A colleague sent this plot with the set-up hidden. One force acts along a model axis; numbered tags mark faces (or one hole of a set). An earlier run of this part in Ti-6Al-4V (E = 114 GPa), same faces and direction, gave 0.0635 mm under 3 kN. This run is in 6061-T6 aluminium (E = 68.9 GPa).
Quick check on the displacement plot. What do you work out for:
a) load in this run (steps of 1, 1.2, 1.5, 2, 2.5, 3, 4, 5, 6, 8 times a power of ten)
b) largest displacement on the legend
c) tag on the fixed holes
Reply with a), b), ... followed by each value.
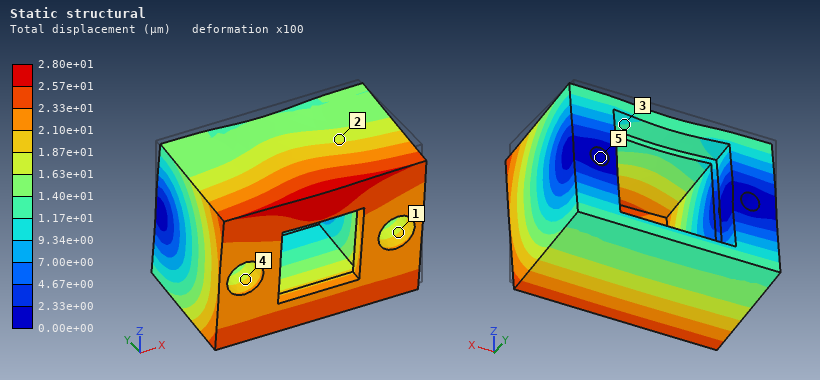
a) 800 N
b) 2.80e+01 µm
c) 5
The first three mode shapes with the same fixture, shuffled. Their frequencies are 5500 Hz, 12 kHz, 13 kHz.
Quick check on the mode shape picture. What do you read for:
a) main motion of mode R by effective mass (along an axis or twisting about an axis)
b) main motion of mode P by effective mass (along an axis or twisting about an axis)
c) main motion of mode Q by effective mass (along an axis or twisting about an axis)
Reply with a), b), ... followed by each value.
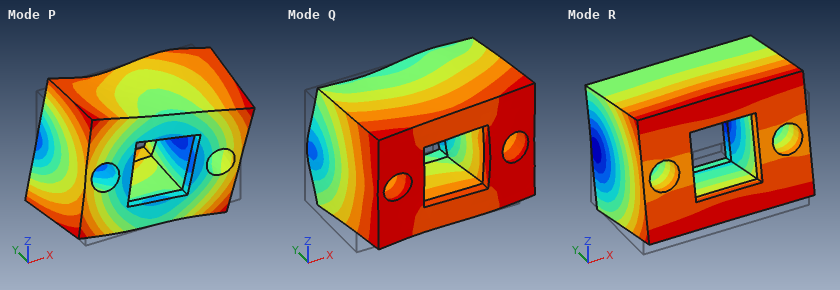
a) along Z
b) twisting about Y
c) along X
